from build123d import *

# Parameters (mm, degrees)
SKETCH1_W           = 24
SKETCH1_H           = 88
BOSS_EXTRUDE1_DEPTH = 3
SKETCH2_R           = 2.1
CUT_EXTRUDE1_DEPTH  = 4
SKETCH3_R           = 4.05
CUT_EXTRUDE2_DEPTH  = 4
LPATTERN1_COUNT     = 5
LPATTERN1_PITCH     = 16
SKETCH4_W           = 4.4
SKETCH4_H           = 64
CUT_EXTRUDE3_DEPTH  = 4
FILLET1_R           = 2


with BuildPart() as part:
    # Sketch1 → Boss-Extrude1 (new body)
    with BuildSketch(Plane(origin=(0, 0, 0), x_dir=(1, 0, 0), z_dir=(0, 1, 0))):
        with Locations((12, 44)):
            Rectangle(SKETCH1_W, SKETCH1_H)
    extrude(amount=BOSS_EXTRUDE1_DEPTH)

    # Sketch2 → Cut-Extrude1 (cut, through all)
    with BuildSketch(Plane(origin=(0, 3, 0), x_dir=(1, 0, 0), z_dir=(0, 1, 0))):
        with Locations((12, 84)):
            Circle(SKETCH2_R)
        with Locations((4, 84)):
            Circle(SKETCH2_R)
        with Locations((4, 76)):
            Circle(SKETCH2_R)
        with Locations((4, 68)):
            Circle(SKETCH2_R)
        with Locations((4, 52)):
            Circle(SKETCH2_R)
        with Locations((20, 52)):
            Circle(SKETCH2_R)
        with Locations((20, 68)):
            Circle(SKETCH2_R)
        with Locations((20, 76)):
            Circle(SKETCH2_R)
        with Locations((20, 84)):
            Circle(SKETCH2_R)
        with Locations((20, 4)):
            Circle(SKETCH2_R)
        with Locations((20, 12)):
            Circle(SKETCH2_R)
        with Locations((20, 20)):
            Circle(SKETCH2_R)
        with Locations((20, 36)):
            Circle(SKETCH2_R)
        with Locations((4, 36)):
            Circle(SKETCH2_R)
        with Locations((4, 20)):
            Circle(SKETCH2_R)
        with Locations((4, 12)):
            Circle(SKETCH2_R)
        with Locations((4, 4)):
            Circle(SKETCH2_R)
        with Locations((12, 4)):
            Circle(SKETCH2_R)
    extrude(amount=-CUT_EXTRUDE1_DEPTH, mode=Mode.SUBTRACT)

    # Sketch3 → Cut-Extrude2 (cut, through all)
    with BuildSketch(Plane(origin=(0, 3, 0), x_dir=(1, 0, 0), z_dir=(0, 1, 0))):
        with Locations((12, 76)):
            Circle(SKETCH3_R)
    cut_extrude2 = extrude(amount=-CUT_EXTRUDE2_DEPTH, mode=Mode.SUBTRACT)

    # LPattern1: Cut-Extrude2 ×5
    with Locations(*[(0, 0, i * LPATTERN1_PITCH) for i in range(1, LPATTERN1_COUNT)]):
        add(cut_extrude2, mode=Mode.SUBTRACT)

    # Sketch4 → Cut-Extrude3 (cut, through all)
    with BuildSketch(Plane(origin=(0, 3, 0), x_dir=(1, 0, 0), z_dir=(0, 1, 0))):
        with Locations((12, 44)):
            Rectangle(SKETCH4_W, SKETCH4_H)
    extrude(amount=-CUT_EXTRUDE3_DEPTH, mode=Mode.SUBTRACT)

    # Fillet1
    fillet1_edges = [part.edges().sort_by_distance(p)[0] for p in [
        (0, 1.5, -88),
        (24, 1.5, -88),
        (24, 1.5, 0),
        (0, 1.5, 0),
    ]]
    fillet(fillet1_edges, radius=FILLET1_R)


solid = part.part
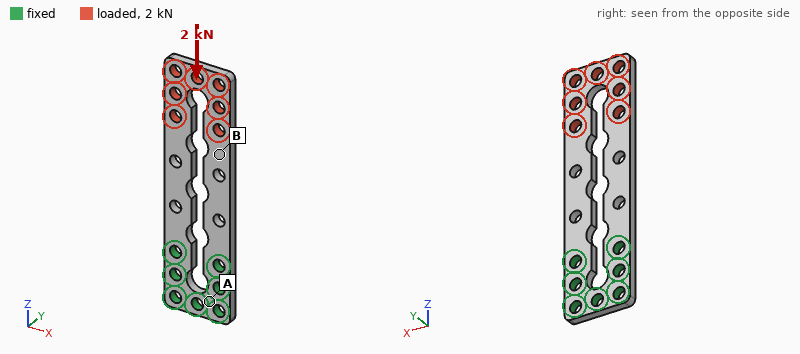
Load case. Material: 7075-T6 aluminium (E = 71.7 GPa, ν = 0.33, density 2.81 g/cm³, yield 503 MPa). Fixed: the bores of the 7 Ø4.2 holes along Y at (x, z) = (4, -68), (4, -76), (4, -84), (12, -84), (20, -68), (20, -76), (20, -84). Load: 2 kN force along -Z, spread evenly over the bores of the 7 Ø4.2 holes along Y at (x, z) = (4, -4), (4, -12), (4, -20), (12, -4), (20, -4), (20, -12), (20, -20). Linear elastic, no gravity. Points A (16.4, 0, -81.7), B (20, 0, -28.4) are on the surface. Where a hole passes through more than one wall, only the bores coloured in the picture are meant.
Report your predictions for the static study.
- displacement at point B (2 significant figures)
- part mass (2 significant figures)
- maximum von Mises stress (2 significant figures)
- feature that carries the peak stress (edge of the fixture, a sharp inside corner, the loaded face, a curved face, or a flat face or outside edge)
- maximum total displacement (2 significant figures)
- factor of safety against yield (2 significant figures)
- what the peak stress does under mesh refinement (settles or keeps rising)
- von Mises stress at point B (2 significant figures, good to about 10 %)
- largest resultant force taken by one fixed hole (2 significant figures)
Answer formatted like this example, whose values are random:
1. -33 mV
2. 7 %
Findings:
1. 28 µm
2. 12 g
3. 170 MPa
4. a curved face
5. 43 µm
6. 2.9
7. settles
8. 27 MPa
9. 930 N
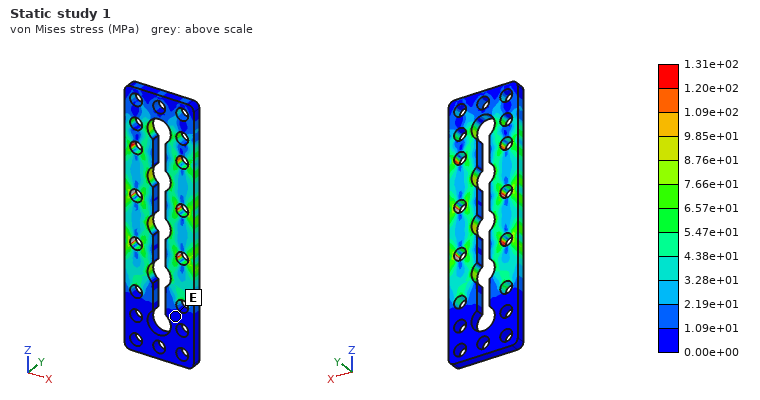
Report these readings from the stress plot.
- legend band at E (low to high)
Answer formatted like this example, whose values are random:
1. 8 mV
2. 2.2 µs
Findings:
1. 0.00e+00 to 1.09e+01 MPa
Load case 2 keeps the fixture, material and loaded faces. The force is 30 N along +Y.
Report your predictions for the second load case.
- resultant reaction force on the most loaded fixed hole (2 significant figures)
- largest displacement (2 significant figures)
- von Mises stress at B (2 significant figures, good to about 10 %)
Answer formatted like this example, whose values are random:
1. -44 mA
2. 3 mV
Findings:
1. 23 N
2. 0.91 mm
3. 21 MPa
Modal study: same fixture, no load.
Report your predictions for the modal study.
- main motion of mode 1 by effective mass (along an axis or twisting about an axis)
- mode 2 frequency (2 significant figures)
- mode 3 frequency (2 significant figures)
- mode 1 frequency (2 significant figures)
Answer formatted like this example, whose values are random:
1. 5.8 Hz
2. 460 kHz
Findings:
1. along Y
2. 2200 Hz
3. 2300 Hz
4. 530 Hz
